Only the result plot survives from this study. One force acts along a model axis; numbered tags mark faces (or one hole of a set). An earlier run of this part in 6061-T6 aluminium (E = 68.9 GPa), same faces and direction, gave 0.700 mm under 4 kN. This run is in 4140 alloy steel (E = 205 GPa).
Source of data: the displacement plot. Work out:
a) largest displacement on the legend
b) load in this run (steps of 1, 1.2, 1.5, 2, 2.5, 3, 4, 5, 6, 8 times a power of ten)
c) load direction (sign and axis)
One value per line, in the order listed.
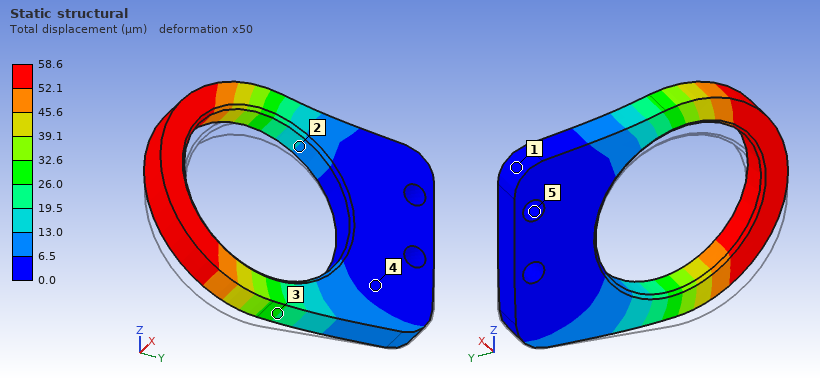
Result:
58.6 µm
1 kN
+Z
